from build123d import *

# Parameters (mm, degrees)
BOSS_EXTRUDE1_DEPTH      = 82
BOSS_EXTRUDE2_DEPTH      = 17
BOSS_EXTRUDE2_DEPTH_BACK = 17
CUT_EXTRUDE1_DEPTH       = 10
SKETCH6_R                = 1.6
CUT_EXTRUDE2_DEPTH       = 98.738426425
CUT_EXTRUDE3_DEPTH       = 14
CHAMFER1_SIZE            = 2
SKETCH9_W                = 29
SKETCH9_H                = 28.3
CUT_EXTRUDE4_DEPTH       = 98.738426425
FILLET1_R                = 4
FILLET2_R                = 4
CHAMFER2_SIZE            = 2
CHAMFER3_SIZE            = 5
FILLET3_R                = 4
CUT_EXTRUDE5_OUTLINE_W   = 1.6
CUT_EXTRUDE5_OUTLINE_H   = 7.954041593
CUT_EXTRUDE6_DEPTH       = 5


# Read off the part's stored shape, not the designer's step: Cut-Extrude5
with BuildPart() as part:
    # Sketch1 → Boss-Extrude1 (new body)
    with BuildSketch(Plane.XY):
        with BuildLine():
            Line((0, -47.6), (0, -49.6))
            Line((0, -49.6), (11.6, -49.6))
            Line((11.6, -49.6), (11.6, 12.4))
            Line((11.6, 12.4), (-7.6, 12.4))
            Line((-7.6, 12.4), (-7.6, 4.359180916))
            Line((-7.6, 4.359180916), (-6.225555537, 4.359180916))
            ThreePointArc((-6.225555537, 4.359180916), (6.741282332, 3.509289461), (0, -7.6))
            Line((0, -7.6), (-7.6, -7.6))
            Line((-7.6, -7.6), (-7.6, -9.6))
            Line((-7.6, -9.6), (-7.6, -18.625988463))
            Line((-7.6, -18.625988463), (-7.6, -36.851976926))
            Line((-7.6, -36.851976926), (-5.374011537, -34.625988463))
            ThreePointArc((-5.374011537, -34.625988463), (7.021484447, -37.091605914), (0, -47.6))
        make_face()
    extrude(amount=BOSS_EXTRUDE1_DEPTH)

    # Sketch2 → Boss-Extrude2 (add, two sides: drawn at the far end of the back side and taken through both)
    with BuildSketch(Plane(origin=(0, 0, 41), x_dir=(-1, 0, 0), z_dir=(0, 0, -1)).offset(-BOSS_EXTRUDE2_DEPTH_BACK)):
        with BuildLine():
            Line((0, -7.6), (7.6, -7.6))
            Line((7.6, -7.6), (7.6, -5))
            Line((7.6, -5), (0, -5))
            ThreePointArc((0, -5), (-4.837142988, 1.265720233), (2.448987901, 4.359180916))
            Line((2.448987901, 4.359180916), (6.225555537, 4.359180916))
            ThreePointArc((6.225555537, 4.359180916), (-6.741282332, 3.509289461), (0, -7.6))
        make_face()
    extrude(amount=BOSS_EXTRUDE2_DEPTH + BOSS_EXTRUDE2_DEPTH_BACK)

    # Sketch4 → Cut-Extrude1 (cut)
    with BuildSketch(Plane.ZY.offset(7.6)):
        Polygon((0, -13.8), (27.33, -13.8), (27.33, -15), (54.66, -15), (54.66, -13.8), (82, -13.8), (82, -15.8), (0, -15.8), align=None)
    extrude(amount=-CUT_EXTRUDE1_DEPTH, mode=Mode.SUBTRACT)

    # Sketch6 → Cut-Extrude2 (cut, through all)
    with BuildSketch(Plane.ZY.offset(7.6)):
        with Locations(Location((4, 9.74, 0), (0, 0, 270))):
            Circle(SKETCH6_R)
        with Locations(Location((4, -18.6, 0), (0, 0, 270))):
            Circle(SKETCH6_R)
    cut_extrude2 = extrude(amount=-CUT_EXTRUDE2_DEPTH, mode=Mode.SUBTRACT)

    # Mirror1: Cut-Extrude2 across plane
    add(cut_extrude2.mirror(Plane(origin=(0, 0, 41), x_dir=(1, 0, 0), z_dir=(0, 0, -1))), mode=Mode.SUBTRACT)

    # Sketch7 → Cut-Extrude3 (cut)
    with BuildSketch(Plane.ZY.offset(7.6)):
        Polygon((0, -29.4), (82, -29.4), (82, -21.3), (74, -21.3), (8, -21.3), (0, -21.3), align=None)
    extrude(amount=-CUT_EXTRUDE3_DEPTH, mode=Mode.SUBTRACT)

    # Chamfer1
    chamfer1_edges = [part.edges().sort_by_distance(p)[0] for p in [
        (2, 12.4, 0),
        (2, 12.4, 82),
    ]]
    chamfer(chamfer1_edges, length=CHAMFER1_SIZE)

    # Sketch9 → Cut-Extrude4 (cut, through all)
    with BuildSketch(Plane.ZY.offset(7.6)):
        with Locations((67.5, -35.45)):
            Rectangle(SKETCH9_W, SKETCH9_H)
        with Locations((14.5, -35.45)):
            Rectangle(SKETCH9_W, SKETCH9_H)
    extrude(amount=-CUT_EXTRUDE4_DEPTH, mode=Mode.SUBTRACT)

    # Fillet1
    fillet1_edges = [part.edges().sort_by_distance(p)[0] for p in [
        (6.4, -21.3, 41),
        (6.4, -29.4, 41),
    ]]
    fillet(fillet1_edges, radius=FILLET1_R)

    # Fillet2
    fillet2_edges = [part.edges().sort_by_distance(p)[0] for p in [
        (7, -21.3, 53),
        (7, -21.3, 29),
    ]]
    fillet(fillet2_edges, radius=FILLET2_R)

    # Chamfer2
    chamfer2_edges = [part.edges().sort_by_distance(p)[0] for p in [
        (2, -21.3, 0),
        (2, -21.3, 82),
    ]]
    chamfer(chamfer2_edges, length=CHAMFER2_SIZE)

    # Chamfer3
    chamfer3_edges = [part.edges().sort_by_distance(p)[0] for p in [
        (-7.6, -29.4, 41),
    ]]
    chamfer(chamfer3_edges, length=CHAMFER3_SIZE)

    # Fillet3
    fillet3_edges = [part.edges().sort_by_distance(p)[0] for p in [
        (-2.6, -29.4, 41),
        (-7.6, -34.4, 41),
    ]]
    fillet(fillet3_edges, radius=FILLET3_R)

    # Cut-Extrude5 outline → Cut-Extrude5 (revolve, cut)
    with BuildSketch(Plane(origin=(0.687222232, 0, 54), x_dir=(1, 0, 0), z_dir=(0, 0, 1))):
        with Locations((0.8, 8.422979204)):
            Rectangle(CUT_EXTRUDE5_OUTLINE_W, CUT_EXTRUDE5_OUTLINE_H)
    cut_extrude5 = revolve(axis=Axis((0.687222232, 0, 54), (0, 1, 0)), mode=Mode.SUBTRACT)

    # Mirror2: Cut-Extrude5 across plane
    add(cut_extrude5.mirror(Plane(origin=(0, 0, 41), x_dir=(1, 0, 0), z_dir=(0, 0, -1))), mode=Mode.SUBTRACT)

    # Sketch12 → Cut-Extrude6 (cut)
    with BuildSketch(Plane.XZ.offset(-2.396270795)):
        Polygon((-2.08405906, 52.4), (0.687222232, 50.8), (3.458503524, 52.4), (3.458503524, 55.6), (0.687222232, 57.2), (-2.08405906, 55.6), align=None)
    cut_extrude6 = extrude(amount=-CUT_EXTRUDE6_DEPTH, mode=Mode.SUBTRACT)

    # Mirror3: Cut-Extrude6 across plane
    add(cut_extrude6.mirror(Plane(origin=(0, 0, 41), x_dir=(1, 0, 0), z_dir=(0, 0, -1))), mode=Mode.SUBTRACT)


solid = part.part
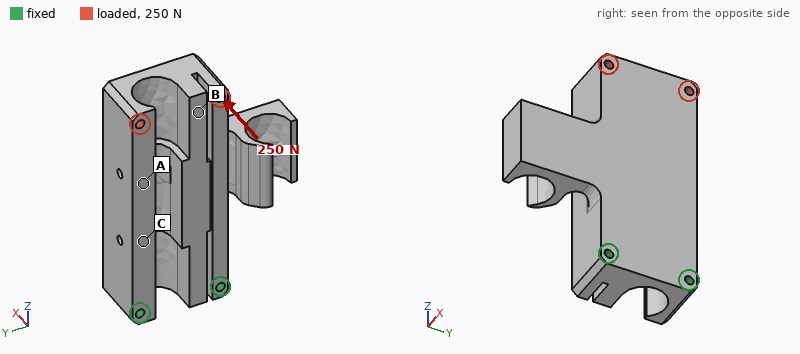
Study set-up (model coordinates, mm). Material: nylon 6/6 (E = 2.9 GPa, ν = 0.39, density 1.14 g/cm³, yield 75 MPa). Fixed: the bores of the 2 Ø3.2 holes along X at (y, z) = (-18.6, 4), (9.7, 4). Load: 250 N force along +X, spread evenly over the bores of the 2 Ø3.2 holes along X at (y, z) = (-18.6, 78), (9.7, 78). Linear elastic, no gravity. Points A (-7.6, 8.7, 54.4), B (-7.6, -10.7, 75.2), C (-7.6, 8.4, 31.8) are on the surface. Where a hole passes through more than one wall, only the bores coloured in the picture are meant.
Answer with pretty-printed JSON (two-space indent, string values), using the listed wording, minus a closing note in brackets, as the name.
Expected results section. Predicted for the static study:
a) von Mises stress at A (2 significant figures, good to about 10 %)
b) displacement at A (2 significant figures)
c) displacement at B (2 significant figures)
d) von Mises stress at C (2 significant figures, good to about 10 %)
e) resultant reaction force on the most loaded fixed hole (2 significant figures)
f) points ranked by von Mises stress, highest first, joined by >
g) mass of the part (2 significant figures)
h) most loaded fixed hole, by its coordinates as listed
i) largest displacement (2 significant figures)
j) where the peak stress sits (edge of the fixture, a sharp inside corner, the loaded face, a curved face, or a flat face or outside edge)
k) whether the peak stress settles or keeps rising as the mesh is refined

{
  "von Mises stress at A": "4.9 MPa",
  "displacement at A": "0.63 mm",
  "displacement at B": "1.0 mm",
  "von Mises stress at C": "8.8 MPa",
  "resultant reaction force on the most loaded fixed hole": "170 N",
  "points ranked by von Mises stress, highest first, joined by >": "C > A > B",
  "mass of the part": "49 g",
  "most loaded fixed hole, by its coordinates as listed": "(9.7, 4)",
  "largest displacement": "1.2 mm",
  "where the peak stress sits": "edge of the fixture",
  "whether the peak stress settles or keeps rising as the mesh is refined": "keeps rising"
}
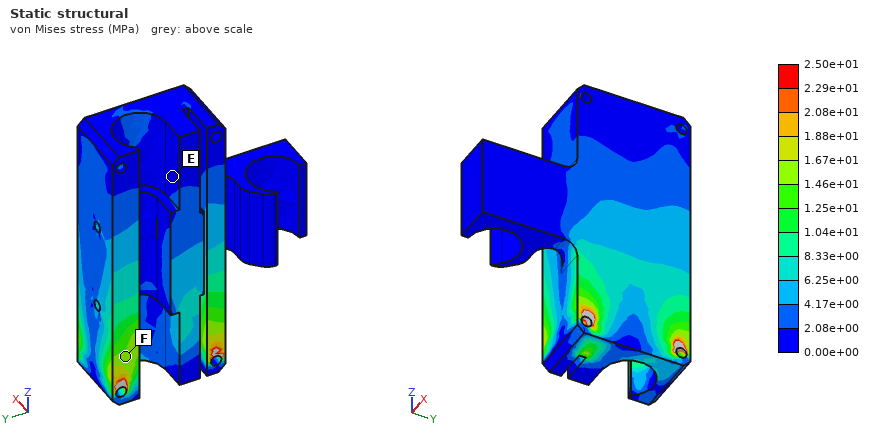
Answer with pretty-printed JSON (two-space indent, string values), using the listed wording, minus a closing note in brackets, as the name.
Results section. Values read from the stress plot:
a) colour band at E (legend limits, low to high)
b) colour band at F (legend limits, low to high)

{
  "colour band at E": "0.00e+00 to 2.08e+00 MPa",
  "colour band at F": "1.46e+01 to 1.67e+01 MPa"
}
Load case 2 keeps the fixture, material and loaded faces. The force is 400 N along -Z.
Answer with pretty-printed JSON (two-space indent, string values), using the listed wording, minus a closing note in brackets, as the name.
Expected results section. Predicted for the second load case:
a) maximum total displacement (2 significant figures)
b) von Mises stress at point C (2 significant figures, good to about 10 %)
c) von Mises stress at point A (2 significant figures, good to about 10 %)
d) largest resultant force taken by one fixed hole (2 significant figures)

{
  "maximum total displacement": "68 µm",
  "von Mises stress at point C": "1.6 MPa",
  "von Mises stress at point A": "1.7 MPa",
  "largest resultant force taken by one fixed hole": "200 N"
}
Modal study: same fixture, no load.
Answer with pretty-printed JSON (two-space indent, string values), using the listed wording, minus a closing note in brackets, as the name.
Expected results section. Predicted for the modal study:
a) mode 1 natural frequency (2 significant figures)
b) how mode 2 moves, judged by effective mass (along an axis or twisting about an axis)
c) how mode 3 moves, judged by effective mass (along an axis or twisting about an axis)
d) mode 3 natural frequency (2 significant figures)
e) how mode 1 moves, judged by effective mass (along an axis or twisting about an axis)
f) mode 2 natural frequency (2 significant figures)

{
  "mode 1 natural frequency": "660 Hz",
  "how mode 2 moves, judged by effective mass": "along Y",
  "how mode 3 moves, judged by effective mass": "along Y",
  "mode 3 natural frequency": "1200 Hz",
  "how mode 1 moves, judged by effective mass": "along X",
  "mode 2 natural frequency": "900 Hz"
}
